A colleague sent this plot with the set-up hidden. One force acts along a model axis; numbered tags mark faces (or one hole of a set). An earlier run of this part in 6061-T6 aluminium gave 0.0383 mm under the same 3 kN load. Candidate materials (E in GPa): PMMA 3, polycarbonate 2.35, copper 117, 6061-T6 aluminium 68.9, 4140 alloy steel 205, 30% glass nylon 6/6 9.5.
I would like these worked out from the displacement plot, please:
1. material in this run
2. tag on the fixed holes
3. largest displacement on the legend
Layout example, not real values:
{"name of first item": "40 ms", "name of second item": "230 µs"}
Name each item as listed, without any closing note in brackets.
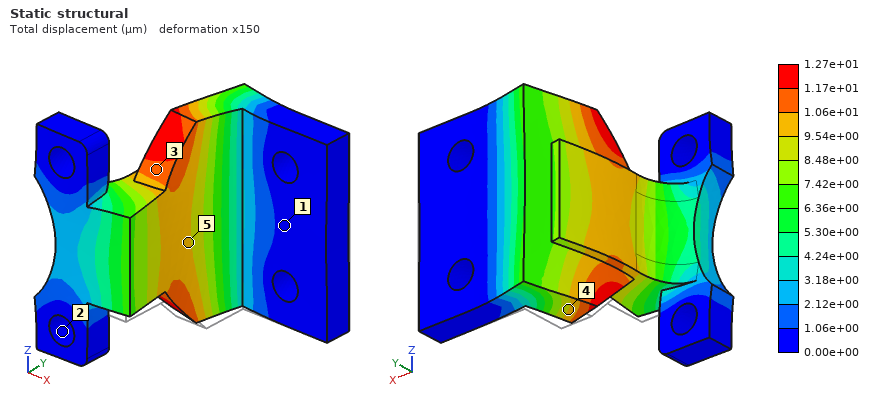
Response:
{"material in this run": "4140 alloy steel", "tag on the fixed holes": "2", "largest displacement on the legend": "1.27e+01 µm"}
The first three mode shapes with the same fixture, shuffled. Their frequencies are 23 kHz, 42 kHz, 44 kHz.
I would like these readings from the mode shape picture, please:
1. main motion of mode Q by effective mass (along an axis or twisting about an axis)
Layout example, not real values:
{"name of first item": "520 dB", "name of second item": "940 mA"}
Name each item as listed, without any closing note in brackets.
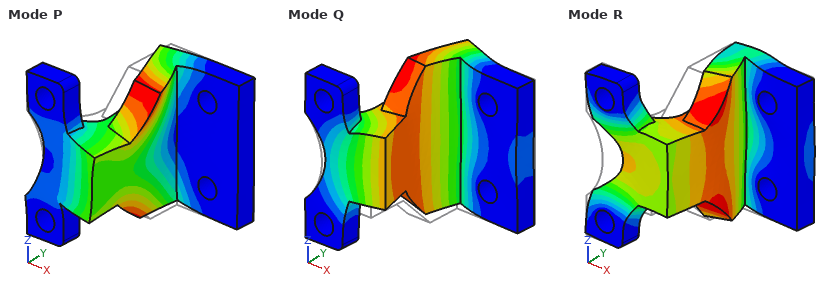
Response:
{"main motion of mode Q by effective mass": "along Y"}
